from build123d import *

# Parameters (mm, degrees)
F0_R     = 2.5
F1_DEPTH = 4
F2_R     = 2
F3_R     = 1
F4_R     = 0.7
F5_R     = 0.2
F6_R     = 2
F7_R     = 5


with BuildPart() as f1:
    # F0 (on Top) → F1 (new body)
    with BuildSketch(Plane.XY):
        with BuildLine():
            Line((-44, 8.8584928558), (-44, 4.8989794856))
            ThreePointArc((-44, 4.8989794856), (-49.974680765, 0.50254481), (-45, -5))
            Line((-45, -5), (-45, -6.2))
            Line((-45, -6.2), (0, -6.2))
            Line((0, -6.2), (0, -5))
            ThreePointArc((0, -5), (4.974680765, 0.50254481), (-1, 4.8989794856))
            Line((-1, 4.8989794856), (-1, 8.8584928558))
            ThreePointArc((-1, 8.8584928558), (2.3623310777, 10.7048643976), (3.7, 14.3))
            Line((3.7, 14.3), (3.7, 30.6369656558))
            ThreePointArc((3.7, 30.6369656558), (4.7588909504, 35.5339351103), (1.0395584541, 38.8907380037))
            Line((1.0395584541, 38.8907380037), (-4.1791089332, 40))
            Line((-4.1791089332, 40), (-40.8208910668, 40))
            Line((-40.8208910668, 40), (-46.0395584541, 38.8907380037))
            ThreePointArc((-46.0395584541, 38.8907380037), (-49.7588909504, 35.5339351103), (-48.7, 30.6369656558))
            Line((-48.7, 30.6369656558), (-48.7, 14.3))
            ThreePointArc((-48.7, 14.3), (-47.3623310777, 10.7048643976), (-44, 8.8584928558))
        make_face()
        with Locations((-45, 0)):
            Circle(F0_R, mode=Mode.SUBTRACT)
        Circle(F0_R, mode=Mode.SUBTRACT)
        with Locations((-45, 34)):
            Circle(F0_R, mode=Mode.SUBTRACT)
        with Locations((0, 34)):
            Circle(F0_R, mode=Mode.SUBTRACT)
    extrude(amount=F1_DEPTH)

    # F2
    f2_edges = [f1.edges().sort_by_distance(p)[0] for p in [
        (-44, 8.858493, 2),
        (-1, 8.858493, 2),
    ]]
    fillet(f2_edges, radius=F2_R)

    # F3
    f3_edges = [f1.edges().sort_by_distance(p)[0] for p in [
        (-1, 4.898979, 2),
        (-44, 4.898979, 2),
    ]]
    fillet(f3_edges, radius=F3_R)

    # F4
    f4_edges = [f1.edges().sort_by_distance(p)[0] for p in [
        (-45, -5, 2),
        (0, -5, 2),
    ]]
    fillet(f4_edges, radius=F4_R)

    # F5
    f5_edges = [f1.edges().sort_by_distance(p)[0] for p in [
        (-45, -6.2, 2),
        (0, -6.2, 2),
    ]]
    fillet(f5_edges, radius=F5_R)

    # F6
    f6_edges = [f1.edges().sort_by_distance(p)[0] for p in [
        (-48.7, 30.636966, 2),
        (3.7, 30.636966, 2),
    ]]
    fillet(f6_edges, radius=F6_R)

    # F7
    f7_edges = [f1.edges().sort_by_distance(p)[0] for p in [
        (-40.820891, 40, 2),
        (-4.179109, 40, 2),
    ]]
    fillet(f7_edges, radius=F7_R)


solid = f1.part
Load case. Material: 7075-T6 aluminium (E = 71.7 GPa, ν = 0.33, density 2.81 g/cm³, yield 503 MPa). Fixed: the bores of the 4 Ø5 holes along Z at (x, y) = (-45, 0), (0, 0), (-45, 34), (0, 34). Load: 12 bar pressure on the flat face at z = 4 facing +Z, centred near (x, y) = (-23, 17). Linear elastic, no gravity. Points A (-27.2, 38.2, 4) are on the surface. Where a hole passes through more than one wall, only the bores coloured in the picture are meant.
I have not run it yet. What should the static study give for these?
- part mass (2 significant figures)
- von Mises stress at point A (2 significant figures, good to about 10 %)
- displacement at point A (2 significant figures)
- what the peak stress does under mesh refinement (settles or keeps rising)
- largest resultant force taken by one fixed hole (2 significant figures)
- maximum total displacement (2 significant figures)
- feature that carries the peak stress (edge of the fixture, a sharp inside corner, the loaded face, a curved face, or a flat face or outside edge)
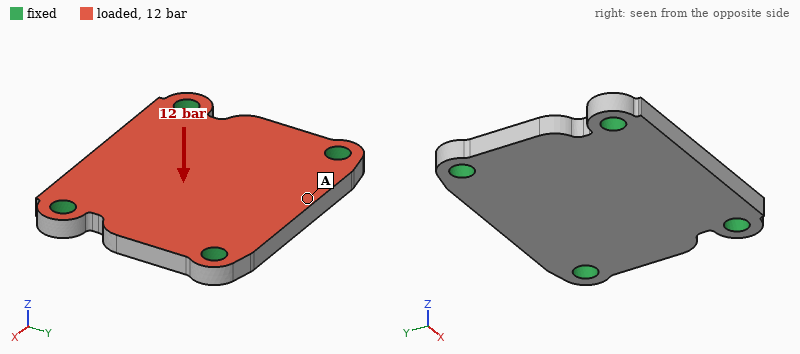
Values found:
26 g
35 MPa
32 µm
keeps rising
700 N
48 µm
edge of the fixture
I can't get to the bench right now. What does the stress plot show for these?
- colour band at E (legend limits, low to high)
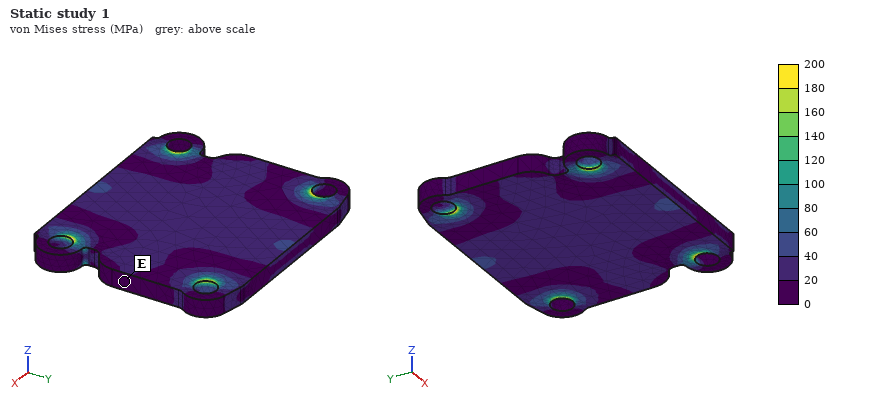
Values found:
0 to 20 MPa
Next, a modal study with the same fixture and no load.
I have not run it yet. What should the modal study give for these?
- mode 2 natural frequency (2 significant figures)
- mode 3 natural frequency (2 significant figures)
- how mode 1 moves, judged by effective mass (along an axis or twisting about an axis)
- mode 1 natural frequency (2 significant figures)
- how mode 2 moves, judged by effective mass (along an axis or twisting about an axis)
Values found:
13 kHz
16 kHz
along Z
9000 Hz
twisting about X
